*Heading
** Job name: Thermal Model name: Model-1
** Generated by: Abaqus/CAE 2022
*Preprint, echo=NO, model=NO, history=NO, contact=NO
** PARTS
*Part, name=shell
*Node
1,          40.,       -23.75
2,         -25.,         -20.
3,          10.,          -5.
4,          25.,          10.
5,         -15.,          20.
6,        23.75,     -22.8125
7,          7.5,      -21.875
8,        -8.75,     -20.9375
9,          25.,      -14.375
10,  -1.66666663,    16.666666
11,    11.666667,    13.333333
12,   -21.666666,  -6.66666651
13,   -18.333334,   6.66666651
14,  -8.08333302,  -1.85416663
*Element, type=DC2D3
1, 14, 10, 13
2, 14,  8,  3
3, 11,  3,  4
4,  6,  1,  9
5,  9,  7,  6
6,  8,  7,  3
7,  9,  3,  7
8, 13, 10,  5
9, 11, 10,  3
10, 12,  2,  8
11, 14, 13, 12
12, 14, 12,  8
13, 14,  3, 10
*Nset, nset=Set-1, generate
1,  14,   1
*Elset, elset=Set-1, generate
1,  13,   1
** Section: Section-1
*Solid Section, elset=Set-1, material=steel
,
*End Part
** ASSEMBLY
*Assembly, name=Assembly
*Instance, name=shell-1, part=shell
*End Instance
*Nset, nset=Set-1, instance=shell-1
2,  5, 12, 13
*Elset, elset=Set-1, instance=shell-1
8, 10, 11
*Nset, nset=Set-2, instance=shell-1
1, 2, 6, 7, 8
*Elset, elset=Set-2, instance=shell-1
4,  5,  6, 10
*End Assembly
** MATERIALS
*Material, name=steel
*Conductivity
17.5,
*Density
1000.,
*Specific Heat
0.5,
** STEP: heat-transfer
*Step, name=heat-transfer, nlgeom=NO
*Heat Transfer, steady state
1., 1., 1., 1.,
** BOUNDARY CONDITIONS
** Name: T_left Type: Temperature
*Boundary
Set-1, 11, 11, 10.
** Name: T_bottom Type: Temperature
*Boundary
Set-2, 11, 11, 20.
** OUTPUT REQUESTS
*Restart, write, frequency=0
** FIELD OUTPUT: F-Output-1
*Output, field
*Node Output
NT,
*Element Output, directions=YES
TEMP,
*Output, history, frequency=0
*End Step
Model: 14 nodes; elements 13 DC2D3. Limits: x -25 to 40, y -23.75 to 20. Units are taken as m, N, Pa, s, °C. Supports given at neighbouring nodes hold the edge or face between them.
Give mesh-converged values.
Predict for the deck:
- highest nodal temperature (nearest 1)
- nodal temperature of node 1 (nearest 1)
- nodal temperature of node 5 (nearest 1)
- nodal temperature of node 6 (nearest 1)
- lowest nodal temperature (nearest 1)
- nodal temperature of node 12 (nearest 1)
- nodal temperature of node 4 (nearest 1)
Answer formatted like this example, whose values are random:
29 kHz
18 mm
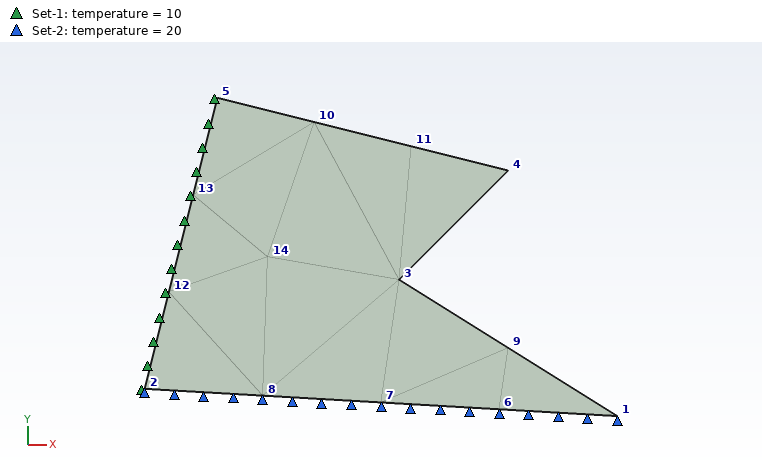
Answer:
20 °C
20 °C
10 °C
20 °C
10 °C
10 °C
15 °C
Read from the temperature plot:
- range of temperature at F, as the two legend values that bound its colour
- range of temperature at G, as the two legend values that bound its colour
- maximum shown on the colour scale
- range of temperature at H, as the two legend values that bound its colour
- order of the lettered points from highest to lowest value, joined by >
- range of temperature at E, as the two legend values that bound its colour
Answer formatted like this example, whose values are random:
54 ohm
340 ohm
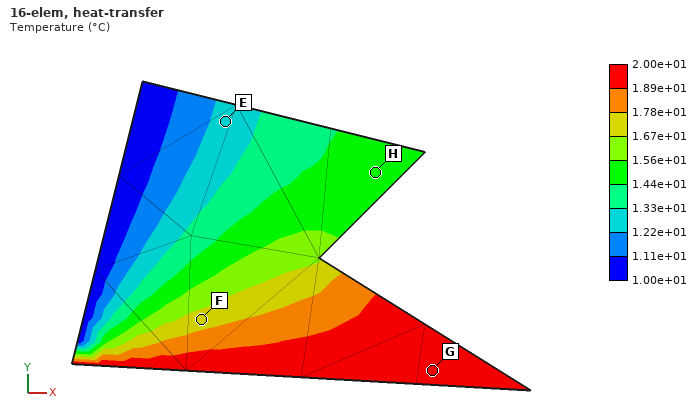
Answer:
1.67e+01 to 1.78e+01 °C
1.89e+01 to 2.00e+01 °C
2.00e+01 °C
1.44e+01 to 1.56e+01 °C
G > F > H > E
1.22e+01 to 1.33e+01 °C
